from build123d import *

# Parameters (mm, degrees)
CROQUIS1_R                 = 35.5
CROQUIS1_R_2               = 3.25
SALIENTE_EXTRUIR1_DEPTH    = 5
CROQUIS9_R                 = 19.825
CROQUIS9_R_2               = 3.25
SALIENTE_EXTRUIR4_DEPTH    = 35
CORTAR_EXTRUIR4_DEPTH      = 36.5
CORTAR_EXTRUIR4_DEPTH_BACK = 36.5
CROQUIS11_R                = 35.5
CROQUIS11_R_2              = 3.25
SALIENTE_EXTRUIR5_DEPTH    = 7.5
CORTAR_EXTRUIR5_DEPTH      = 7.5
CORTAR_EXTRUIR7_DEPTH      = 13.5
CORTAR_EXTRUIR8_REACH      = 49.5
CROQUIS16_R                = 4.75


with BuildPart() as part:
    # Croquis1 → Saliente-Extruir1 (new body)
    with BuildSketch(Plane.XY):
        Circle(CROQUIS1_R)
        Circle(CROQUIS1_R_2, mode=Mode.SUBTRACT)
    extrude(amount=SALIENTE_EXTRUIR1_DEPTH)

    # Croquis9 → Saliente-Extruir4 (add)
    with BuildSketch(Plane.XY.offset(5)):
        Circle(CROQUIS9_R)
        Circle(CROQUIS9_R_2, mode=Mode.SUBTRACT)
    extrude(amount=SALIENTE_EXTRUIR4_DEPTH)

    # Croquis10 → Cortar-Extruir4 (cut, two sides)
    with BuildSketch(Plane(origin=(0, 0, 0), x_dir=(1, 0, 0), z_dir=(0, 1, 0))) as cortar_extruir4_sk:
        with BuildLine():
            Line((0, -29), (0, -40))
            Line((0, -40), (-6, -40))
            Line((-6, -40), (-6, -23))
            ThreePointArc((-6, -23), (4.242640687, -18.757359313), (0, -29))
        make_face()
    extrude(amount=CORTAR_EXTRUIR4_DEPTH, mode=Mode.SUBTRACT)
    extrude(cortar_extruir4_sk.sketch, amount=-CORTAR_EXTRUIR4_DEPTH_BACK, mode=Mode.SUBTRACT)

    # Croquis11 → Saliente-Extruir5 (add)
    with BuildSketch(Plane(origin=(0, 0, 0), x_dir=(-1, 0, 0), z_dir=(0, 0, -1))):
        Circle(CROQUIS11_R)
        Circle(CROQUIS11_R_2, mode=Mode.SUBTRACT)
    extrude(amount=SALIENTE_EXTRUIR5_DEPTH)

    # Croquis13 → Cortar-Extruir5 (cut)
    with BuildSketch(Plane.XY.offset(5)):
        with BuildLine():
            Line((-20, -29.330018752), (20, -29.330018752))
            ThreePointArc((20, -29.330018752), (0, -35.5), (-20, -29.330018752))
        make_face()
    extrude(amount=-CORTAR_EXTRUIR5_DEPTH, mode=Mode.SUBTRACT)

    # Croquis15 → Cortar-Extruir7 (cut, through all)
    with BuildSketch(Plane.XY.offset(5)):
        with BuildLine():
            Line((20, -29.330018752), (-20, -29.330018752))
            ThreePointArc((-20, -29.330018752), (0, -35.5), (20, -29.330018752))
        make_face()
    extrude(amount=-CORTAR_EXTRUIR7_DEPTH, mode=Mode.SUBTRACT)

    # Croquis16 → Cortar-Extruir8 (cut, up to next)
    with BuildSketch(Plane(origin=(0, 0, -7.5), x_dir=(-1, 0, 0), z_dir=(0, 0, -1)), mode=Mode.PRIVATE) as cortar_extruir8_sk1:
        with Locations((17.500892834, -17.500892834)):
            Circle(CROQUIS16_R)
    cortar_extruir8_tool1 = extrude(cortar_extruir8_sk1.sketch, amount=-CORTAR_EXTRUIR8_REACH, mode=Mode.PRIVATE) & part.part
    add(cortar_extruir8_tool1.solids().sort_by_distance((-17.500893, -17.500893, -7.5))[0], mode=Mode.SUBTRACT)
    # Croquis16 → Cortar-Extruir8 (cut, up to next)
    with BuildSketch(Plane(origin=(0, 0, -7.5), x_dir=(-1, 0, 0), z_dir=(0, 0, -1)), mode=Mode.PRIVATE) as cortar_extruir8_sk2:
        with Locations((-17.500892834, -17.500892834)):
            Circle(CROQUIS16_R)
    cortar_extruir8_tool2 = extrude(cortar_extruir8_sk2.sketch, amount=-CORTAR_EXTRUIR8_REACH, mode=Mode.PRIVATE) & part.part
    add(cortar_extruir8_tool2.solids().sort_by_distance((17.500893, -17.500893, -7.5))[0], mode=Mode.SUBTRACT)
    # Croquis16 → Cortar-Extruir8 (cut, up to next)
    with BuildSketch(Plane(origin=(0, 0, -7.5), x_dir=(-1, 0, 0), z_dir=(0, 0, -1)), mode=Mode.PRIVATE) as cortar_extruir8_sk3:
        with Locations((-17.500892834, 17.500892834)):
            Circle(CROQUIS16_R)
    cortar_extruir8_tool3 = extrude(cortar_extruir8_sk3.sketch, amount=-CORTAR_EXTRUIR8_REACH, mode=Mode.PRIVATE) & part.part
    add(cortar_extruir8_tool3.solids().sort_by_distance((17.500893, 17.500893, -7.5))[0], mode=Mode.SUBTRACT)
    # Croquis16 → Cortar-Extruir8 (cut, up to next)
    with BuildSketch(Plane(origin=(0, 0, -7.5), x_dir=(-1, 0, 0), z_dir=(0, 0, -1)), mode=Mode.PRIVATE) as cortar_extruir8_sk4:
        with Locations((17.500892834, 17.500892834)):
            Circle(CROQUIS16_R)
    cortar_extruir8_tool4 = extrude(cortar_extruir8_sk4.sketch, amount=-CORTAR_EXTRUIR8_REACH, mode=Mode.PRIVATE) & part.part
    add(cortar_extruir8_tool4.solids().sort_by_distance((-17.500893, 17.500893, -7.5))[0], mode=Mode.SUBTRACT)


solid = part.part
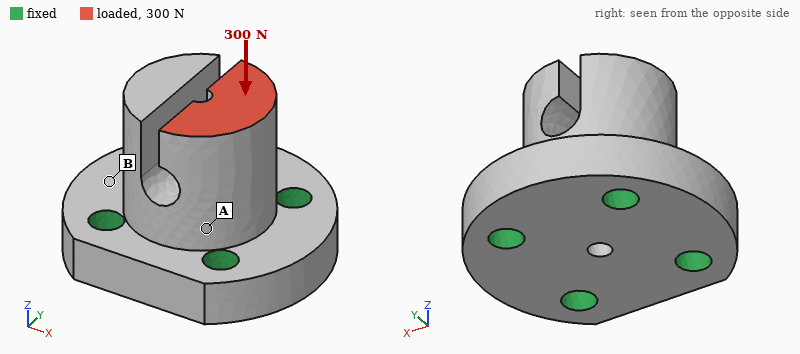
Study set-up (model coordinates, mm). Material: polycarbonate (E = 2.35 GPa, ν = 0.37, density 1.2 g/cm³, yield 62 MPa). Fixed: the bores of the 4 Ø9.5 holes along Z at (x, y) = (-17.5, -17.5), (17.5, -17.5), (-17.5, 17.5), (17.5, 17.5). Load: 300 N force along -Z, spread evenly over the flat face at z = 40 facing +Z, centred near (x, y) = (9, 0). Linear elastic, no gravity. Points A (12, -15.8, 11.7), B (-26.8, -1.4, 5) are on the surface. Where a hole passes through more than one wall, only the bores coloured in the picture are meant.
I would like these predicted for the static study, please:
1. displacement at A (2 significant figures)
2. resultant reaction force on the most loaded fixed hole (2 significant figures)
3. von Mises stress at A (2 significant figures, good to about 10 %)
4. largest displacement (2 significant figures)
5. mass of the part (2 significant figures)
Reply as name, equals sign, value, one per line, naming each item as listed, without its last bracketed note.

displacement at A = 5.3 µm
resultant reaction force on the most loaded fixed hole = 120 N
von Mises stress at A = 0.86 MPa
largest displacement = 27 µm
mass of the part = 95 g
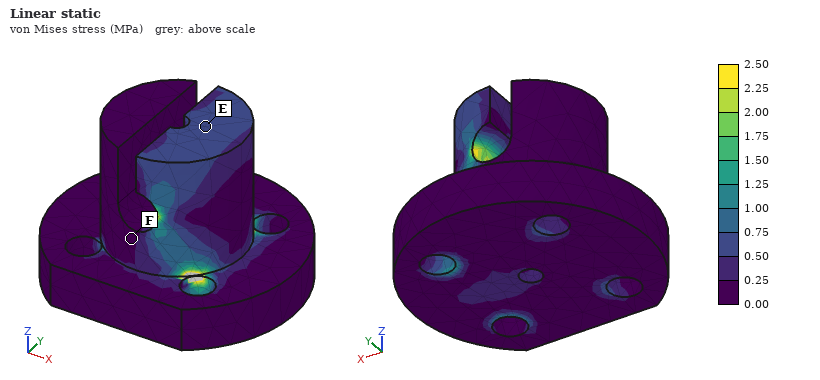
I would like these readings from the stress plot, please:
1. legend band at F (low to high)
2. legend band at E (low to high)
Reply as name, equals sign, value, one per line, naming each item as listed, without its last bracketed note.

legend band at F = 0.00 to 0.25 MPa
legend band at E = 0.50 to 0.75 MPa
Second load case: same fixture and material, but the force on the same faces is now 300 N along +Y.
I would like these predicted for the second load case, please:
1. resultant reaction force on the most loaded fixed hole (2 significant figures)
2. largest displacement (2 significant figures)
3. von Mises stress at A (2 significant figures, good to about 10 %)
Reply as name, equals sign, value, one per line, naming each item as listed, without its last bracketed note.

resultant reaction force on the most loaded fixed hole = 250 N
largest displacement = 0.12 mm
von Mises stress at A = 3.6 MPa
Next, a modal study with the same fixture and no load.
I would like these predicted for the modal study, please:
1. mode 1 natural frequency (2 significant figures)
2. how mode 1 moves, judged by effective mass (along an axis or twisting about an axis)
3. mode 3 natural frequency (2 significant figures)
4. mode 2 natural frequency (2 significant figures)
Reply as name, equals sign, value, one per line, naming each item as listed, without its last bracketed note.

mode 1 natural frequency = 2500 Hz
how mode 1 moves, judged by effective mass = along X
mode 3 natural frequency = 3100 Hz
mode 2 natural frequency = 3100 Hz
